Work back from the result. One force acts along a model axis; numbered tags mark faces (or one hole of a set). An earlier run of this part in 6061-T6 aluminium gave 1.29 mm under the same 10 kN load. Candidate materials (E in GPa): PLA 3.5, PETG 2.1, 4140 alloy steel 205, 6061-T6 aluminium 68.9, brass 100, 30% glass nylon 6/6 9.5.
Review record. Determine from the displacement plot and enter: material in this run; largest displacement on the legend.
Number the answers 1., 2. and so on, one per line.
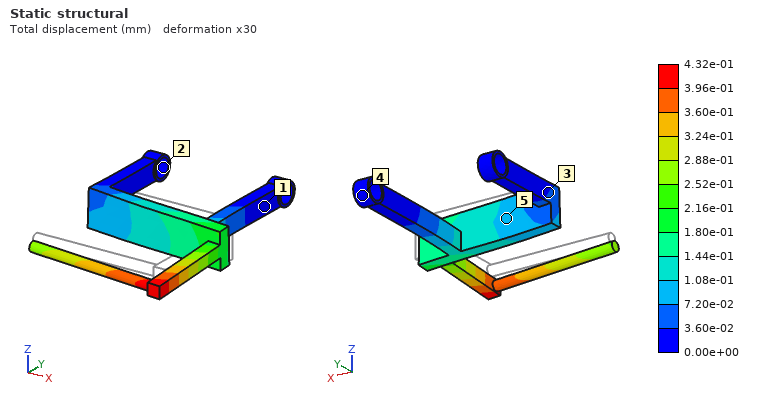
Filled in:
1. 4140 alloy steel
2. 4.32e-01 mm
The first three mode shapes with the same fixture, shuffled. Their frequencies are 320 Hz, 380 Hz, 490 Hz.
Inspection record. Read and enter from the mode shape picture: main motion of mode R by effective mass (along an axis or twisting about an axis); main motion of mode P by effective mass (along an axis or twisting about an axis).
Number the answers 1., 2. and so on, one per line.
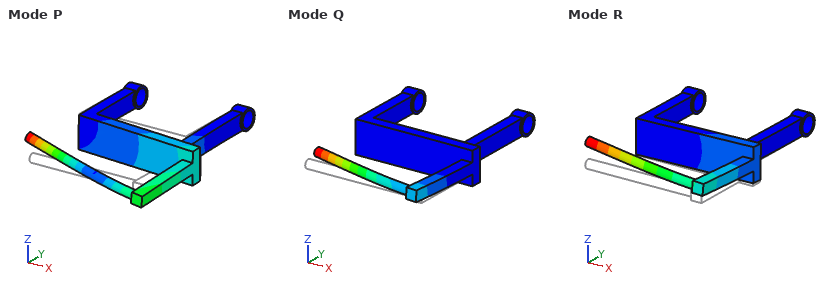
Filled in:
1. along Z
2. along Z
